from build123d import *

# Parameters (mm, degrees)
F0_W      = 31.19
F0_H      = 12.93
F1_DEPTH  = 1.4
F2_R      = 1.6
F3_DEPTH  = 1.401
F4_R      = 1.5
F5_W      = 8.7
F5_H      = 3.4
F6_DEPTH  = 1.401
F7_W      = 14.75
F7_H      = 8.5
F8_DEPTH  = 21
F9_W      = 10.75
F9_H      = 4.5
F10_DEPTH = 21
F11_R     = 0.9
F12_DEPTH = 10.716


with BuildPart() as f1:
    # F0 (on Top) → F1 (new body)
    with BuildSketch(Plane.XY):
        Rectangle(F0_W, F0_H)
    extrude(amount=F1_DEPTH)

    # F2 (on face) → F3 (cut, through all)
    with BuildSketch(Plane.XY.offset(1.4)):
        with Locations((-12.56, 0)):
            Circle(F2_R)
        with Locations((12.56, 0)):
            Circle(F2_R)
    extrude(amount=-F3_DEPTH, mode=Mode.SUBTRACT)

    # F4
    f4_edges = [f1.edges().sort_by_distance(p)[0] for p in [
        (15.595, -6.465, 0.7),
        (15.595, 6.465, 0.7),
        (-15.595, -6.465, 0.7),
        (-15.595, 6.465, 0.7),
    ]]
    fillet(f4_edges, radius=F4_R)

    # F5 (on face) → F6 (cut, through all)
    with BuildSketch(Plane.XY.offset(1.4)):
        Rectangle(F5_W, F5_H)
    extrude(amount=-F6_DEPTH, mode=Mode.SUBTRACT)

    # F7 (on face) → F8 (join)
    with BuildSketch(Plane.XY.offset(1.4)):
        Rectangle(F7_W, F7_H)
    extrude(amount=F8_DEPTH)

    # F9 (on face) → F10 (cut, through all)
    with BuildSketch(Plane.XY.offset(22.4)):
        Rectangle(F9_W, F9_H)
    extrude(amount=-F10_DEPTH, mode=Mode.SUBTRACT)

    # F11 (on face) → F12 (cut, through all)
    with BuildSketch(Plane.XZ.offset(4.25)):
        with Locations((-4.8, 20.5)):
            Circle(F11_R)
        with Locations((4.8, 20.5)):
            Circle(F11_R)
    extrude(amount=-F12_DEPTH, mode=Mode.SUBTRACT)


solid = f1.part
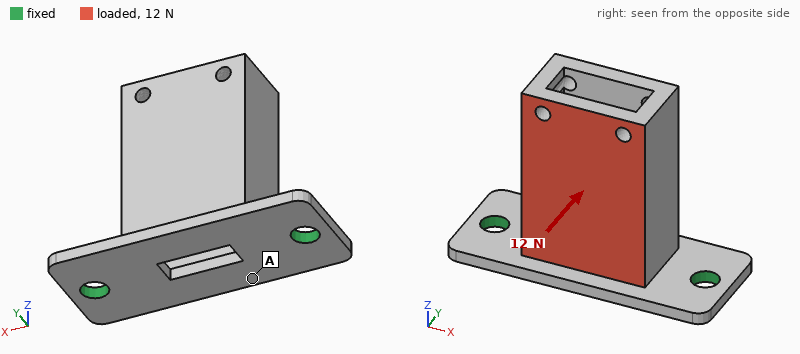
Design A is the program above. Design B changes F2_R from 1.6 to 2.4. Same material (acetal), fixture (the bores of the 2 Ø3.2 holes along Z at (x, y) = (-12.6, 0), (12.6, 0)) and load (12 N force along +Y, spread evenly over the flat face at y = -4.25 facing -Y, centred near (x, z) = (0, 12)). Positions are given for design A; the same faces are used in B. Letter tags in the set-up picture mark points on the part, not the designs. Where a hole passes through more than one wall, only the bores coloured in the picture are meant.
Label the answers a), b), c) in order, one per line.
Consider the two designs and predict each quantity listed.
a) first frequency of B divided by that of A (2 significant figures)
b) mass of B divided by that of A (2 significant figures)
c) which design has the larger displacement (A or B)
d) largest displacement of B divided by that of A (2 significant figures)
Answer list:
a) 1.2
b) 0.99
c) A
d) 0.65
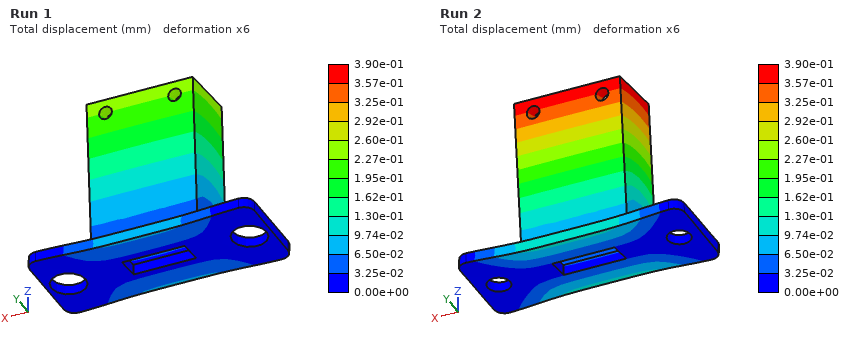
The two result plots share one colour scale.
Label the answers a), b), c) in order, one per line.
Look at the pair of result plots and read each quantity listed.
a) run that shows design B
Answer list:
a) Run 1
